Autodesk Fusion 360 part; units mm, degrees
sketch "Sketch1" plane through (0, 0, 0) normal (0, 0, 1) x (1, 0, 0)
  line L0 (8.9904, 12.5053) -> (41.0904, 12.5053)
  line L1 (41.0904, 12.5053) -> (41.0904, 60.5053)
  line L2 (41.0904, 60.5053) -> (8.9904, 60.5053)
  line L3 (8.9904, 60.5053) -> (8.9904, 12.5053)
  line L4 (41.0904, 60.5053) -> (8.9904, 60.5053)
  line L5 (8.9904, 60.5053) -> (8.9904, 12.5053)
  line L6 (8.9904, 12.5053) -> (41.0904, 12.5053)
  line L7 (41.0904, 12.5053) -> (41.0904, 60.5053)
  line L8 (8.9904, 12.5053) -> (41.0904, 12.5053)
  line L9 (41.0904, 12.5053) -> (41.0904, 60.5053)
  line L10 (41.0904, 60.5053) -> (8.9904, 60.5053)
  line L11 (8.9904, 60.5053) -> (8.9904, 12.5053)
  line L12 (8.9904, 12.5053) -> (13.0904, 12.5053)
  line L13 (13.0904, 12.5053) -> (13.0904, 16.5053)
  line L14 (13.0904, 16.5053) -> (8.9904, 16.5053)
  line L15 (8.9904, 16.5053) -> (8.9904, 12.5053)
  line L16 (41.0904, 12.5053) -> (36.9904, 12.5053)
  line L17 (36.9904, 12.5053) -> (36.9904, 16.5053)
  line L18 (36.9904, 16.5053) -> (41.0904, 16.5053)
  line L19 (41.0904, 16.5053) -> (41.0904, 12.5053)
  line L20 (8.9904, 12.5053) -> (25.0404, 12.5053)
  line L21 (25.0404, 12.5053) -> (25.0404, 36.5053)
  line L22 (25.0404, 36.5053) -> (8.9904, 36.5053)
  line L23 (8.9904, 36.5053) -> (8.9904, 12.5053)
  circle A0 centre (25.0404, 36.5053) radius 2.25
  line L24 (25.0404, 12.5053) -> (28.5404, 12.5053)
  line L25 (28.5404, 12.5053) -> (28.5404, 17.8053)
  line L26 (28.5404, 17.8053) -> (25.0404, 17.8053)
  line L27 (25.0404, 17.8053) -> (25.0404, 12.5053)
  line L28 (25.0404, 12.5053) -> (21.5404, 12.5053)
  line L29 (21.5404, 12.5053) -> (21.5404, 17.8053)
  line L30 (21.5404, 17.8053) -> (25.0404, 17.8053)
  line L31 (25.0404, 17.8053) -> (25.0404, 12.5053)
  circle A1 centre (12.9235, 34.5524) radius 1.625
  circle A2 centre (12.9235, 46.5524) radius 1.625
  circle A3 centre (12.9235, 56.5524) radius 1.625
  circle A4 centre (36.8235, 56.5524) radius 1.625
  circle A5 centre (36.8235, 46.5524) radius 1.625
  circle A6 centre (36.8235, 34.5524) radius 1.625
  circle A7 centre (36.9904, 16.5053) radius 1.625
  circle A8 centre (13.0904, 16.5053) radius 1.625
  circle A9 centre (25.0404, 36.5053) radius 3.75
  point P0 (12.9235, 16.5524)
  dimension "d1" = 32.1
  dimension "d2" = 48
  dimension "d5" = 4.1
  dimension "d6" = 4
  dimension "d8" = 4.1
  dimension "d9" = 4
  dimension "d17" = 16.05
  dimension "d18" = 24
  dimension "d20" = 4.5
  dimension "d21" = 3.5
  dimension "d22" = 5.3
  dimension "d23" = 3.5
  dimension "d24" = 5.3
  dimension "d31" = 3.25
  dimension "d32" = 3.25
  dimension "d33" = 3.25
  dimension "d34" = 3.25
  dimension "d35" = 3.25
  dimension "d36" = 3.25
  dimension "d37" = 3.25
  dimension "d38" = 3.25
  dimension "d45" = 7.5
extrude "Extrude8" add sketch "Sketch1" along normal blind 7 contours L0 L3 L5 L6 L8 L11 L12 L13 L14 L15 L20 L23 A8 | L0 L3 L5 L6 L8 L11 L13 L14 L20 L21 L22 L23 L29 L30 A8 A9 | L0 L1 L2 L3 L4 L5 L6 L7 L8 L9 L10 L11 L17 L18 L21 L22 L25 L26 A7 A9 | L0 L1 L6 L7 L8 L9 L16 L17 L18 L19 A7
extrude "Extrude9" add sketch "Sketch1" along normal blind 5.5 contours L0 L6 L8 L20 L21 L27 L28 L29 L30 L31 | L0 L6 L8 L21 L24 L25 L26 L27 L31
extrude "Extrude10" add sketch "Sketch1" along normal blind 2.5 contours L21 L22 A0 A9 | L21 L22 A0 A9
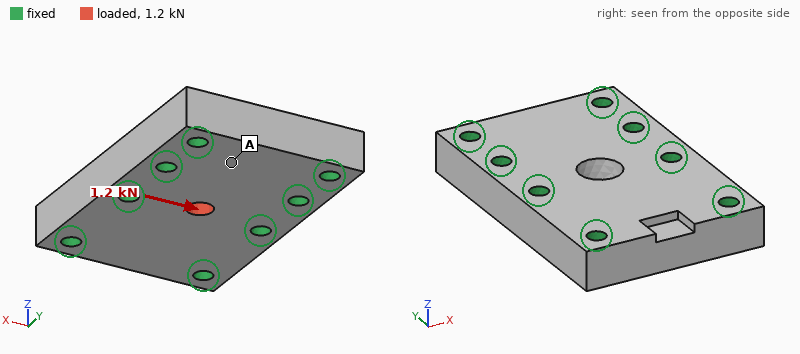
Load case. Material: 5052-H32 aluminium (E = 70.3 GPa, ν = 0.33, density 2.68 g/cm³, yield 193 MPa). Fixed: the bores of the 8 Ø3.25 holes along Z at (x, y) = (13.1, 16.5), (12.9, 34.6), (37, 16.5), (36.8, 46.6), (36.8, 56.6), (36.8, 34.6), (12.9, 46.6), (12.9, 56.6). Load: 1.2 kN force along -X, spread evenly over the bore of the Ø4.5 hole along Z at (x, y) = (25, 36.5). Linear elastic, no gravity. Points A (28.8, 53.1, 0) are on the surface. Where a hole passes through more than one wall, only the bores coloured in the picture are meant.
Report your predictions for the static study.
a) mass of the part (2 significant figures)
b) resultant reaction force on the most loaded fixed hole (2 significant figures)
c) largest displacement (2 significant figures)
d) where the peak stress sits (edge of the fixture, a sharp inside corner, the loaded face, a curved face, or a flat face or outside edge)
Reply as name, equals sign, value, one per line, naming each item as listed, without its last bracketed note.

mass of the part = 27 g
resultant reaction force on the most loaded fixed hole = 390 N
largest displacement = 2.7 µm
where the peak stress sits = the loaded face
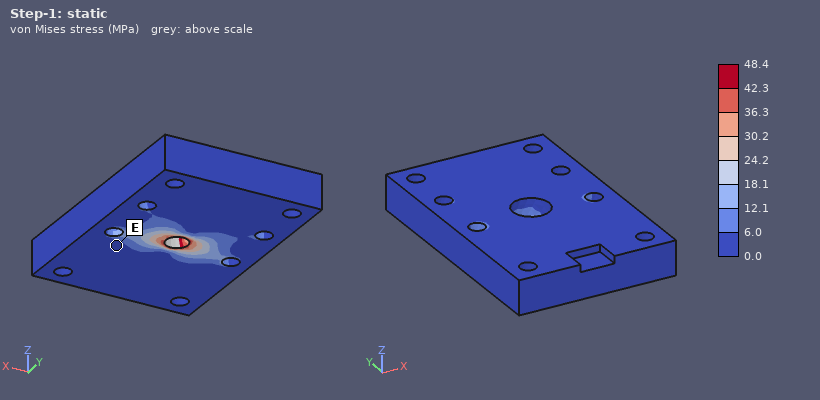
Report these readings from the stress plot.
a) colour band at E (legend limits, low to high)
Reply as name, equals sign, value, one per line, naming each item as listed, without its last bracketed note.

colour band at E = 0.0 to 6.0 MPa
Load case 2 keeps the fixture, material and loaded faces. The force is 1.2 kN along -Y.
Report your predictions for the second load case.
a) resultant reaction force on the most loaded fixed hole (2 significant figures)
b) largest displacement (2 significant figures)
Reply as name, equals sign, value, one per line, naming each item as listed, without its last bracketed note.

resultant reaction force on the most loaded fixed hole = 220 N
largest displacement = 3.1 µm
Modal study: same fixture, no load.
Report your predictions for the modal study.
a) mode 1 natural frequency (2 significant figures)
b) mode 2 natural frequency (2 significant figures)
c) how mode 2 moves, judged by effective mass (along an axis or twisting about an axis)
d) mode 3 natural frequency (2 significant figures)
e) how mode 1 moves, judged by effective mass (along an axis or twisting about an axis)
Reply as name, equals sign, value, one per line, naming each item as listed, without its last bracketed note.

mode 1 natural frequency = 41 kHz
mode 2 natural frequency = 48 kHz
how mode 2 moves, judged by effective mass = along Z
mode 3 natural frequency = 56 kHz
how mode 1 moves, judged by effective mass = along Z
